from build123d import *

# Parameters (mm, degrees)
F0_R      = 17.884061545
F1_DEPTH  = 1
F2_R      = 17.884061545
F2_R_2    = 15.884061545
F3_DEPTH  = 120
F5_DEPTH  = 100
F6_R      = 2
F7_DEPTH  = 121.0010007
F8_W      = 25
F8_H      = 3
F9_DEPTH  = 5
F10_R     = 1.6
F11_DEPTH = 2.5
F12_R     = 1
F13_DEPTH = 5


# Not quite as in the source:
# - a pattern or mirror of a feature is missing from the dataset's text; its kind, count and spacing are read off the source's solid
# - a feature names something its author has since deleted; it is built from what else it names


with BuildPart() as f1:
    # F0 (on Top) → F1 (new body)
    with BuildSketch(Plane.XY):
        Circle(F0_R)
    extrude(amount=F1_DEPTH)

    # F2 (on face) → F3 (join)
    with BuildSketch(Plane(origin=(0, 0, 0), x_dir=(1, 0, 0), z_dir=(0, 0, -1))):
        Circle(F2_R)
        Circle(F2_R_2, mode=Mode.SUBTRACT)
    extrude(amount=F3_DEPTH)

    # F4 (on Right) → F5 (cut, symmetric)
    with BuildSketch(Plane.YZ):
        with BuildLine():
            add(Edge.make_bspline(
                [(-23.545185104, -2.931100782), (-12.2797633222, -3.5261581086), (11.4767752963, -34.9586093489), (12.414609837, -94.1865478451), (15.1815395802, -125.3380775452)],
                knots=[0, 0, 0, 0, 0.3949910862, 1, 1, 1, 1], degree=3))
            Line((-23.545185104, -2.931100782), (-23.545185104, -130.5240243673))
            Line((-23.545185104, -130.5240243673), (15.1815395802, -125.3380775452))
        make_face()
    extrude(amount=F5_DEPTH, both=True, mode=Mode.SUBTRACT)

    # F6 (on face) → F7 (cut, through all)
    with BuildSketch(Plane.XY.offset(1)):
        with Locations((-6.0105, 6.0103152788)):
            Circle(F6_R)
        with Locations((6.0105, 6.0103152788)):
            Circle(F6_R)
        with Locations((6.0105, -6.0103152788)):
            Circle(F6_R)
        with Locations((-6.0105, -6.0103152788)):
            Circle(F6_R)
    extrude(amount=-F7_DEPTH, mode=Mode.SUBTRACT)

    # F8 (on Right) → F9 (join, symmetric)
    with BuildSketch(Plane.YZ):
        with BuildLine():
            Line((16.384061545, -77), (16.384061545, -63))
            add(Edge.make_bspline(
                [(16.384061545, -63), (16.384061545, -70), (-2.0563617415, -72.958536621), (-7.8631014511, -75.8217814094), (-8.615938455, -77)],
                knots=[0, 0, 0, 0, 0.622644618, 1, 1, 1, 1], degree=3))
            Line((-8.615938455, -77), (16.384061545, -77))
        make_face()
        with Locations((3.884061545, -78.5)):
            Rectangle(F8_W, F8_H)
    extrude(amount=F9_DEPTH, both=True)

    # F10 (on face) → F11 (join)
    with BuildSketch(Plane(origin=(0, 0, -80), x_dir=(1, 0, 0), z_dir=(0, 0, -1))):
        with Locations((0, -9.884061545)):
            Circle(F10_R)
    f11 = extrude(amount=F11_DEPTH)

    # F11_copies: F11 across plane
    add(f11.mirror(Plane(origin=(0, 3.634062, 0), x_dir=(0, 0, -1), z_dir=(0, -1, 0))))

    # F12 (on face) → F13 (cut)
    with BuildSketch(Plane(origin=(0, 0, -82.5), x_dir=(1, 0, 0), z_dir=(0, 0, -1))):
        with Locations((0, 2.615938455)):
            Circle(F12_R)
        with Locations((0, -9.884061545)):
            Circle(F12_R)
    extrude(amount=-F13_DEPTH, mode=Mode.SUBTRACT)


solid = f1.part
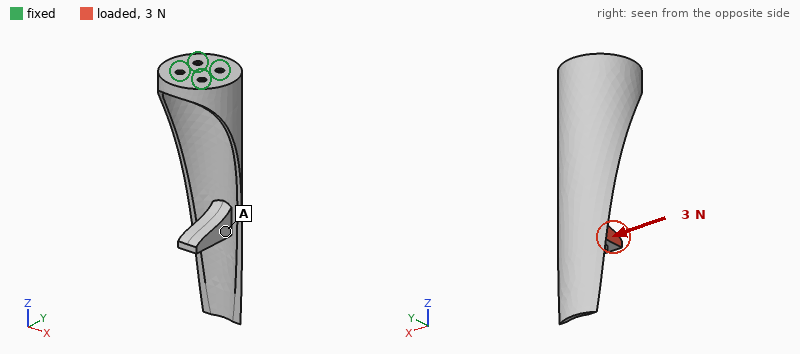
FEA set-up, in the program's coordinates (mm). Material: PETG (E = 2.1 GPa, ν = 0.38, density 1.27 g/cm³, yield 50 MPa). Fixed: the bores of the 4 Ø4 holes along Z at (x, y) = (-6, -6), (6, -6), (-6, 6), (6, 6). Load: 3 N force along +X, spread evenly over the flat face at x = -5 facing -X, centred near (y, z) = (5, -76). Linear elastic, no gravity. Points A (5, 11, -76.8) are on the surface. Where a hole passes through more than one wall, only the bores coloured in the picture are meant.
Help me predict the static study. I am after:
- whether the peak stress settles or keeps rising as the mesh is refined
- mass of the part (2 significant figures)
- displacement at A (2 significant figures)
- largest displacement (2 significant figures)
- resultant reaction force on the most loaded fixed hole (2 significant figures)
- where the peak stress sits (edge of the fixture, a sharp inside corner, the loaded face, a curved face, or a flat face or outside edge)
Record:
keeps rising
16 g
0.77 mm
1.2 mm
7.8 N
edge of the fixture
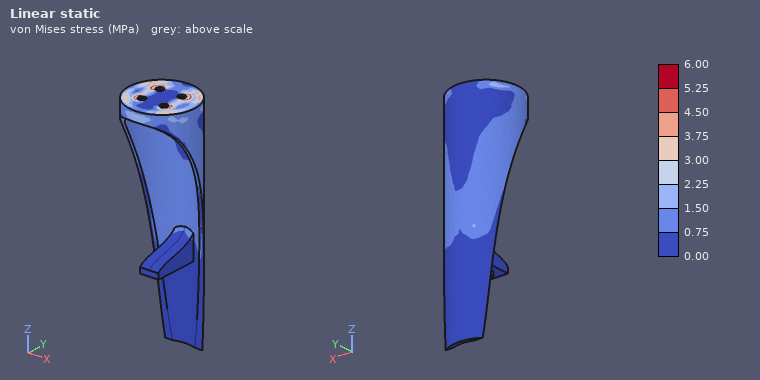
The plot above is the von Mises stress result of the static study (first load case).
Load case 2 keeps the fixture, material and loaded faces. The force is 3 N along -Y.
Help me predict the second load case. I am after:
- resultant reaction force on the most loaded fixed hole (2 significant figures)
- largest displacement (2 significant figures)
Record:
6.9 N
1.2 mm
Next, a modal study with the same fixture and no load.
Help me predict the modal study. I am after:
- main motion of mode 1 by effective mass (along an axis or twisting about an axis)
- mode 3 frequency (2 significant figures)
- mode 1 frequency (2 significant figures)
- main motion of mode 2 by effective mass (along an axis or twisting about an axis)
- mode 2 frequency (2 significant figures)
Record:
along Y
390 Hz
110 Hz
along X
110 Hz
